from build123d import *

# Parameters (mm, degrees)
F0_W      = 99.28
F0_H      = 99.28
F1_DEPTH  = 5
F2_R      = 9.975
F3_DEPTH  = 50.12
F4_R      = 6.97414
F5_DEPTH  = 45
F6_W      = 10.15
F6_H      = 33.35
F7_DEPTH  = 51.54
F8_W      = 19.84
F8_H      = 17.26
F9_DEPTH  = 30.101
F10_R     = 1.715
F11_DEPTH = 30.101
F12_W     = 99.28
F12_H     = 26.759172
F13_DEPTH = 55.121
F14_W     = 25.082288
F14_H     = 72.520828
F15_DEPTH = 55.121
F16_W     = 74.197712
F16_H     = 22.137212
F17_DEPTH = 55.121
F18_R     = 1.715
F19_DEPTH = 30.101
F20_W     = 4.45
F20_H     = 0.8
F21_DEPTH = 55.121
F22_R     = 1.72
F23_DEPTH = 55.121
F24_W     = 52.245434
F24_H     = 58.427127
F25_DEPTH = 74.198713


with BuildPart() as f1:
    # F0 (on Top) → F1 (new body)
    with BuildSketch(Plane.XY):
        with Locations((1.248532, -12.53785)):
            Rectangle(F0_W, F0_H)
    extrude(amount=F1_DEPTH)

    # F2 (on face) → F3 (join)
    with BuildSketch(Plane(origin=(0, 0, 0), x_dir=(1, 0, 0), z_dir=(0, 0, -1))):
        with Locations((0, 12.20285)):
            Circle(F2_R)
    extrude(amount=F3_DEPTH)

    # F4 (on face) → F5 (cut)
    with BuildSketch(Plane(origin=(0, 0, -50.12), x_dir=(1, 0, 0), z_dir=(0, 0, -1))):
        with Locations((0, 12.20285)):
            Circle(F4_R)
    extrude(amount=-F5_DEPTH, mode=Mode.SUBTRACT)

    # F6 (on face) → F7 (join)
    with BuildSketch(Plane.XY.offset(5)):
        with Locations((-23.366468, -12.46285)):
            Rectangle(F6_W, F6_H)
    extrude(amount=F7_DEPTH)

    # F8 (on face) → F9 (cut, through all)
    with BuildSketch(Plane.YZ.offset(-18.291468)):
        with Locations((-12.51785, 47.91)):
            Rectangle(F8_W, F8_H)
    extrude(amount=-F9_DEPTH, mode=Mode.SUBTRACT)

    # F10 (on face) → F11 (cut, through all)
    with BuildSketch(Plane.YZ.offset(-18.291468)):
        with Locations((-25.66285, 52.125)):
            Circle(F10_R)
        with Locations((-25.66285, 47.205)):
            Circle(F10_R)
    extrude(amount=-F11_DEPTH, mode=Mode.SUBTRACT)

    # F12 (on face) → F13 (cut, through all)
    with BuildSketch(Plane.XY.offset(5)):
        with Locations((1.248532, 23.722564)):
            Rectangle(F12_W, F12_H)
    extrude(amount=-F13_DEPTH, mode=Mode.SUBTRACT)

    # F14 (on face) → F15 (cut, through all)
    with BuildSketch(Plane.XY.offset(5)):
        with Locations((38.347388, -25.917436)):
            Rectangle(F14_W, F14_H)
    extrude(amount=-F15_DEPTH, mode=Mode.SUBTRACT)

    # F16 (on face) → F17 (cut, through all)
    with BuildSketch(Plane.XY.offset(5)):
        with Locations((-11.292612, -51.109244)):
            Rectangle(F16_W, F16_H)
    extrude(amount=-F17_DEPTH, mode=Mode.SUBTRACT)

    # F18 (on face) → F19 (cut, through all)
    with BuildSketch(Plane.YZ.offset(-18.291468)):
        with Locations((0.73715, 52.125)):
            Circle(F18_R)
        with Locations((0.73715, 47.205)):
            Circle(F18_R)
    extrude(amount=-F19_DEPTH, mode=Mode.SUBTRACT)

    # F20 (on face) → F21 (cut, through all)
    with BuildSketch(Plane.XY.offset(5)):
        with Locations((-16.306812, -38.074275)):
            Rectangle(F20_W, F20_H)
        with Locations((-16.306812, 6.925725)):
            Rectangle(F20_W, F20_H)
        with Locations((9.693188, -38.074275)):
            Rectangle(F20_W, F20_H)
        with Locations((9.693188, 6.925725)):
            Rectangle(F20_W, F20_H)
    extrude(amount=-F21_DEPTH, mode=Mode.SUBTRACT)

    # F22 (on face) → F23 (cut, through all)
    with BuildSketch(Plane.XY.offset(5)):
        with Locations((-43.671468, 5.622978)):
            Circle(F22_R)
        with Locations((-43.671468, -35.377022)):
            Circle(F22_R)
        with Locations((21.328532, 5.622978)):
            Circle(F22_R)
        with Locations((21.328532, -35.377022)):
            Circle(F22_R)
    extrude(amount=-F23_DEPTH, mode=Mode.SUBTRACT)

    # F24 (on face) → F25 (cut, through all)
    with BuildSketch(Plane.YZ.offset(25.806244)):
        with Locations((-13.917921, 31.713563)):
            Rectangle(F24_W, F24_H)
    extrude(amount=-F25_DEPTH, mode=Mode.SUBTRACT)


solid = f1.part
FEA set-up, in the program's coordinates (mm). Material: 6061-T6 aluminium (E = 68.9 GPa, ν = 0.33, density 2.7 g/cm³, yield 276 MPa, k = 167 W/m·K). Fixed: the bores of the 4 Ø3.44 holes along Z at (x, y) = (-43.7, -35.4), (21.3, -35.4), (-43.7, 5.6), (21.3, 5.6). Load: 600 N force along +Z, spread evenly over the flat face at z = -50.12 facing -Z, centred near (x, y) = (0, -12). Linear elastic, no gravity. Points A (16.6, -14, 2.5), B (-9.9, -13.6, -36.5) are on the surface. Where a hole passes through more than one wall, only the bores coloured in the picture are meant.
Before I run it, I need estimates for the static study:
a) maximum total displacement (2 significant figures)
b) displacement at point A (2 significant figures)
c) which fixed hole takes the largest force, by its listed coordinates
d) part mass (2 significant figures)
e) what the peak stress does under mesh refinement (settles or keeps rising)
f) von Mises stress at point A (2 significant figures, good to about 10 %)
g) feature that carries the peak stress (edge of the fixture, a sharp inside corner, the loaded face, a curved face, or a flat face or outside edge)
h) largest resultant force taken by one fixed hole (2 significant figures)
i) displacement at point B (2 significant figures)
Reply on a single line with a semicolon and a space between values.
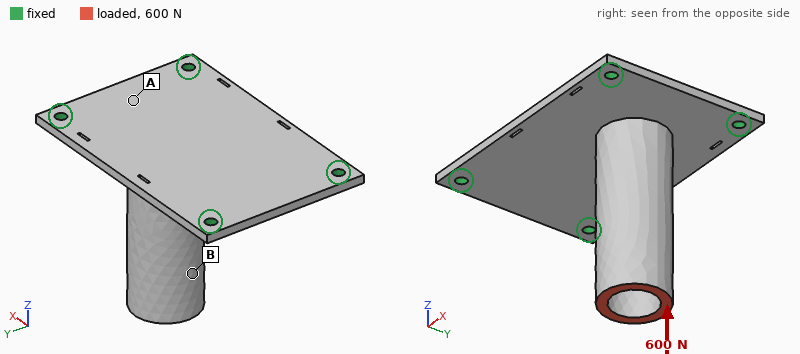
0.25 mm; 0.061 mm; (21.3, 5.6); 49 g; keeps rising; 29 MPa; edge of the fixture; 250 N; 0.21 mm
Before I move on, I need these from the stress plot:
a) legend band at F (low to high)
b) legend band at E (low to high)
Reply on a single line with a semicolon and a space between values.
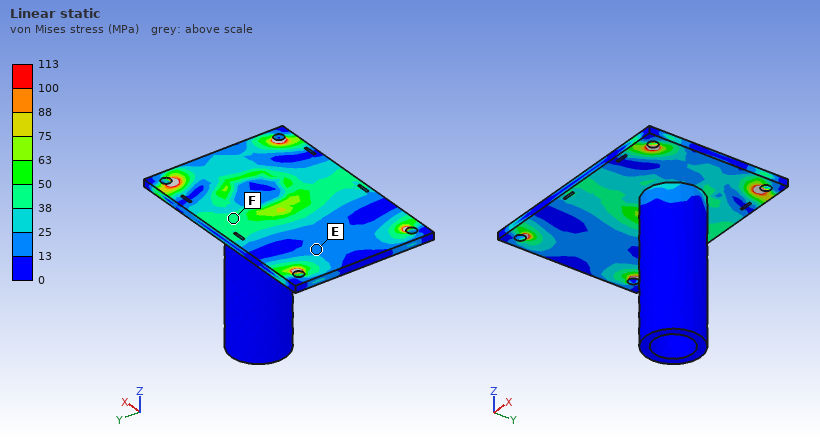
38 to 50 MPa; 13 to 25 MPa
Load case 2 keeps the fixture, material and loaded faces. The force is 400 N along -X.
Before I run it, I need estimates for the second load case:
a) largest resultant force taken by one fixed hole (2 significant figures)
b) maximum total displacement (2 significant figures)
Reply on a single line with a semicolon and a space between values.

250 N; 0.81 mm
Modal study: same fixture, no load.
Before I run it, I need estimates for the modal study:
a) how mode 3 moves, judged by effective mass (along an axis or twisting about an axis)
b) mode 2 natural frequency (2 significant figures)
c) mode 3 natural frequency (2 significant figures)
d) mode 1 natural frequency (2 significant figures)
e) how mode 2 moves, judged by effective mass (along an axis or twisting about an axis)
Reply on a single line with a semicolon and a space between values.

along Z; 1300 Hz; 2300 Hz; 1200 Hz; along Y
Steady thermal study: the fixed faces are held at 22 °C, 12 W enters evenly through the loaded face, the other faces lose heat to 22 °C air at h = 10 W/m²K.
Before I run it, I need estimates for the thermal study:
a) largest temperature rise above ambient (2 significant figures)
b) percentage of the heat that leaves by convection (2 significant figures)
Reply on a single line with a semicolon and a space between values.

30 K; 12 %
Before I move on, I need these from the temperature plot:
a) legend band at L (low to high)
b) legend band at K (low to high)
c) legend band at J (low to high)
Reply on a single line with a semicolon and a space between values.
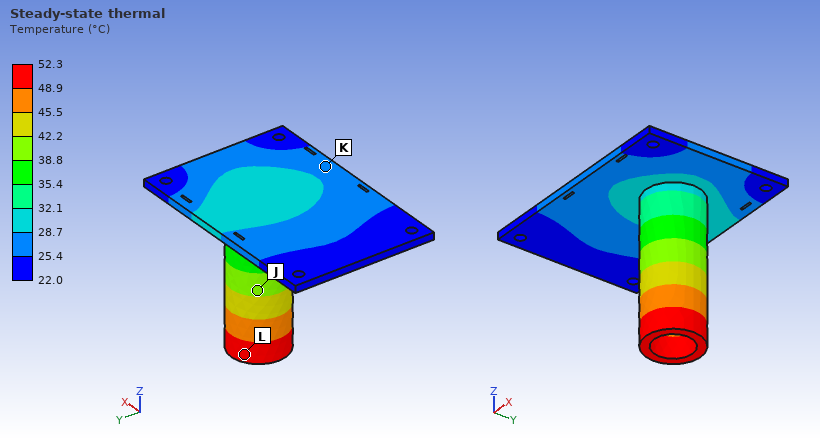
48.9 to 52.3 °C; 25.4 to 28.7 °C; 38.8 to 42.2 °C
